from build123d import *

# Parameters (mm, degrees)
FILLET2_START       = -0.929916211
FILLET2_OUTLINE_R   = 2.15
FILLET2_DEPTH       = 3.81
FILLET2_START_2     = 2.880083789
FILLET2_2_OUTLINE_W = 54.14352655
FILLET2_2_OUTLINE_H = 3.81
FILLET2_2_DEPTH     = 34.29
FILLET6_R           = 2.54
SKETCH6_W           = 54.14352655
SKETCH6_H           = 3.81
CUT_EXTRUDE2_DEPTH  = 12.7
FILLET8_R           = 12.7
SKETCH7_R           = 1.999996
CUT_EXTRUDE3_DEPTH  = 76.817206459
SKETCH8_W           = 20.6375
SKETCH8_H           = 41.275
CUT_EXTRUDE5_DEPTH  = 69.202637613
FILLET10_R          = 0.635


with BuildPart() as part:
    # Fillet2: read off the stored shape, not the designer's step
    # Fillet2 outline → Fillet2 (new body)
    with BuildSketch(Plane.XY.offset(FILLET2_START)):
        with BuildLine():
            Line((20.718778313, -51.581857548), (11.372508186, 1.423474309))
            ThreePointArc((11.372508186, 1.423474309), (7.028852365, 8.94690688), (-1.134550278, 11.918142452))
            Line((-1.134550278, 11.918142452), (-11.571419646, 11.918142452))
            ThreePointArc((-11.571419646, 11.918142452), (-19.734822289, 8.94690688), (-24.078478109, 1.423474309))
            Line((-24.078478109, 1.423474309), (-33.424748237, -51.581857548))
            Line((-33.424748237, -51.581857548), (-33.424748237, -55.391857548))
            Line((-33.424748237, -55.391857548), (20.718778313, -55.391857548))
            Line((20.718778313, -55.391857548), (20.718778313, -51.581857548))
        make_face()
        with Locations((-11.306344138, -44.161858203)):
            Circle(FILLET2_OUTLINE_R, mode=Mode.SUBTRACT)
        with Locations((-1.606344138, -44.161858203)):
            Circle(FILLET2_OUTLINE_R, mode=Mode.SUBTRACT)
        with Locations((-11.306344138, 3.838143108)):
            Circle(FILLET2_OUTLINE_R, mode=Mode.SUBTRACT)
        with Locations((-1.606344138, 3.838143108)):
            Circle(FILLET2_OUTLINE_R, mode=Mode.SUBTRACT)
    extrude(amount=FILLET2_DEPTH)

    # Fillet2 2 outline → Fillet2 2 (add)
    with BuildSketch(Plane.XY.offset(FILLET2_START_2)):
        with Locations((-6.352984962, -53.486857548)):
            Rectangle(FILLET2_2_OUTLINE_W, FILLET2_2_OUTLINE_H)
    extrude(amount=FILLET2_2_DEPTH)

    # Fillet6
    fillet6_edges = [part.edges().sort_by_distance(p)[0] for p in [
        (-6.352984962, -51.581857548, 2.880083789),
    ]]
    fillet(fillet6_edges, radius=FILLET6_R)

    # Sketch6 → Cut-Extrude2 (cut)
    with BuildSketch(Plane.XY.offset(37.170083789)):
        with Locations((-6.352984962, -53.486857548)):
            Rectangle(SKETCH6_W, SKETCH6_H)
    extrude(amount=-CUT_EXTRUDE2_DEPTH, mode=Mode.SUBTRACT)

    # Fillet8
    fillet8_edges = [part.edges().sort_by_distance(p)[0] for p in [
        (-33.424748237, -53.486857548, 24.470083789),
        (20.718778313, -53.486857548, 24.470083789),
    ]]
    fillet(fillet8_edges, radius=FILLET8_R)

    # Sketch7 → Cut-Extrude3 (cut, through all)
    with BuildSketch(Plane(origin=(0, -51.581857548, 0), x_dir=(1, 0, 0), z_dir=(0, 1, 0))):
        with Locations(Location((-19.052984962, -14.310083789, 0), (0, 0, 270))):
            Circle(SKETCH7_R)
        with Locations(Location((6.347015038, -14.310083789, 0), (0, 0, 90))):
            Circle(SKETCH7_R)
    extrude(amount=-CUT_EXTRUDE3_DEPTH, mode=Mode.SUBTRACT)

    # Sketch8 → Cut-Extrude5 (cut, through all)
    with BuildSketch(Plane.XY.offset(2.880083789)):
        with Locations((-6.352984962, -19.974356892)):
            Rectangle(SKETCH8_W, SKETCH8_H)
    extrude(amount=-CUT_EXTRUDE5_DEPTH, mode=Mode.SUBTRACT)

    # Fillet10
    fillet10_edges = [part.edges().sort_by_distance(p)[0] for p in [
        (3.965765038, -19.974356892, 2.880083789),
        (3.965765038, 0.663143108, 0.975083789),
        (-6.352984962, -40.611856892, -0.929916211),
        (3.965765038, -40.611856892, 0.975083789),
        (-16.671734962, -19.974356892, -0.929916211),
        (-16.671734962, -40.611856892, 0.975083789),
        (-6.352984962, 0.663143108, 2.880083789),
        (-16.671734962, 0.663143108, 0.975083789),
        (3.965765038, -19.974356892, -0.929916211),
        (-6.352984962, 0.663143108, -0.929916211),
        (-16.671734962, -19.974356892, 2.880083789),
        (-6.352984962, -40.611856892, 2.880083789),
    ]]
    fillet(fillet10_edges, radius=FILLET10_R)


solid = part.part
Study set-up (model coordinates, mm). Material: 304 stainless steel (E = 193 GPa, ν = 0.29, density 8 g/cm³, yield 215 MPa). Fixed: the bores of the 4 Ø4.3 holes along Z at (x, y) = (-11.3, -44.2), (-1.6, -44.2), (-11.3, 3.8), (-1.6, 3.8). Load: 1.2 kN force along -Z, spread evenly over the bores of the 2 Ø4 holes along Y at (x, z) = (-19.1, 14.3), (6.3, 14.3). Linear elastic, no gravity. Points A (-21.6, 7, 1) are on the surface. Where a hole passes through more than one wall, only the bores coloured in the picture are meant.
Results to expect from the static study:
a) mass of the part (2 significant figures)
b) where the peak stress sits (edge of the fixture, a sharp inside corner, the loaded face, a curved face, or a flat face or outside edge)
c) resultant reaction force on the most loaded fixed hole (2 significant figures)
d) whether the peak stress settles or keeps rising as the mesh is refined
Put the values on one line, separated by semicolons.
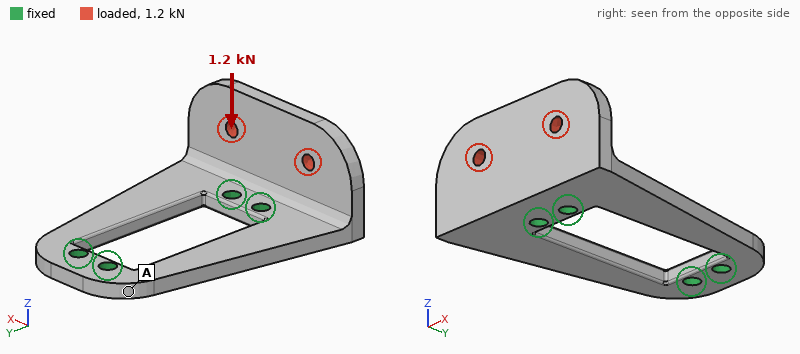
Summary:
93 g; edge of the fixture; 620 N; keeps rising
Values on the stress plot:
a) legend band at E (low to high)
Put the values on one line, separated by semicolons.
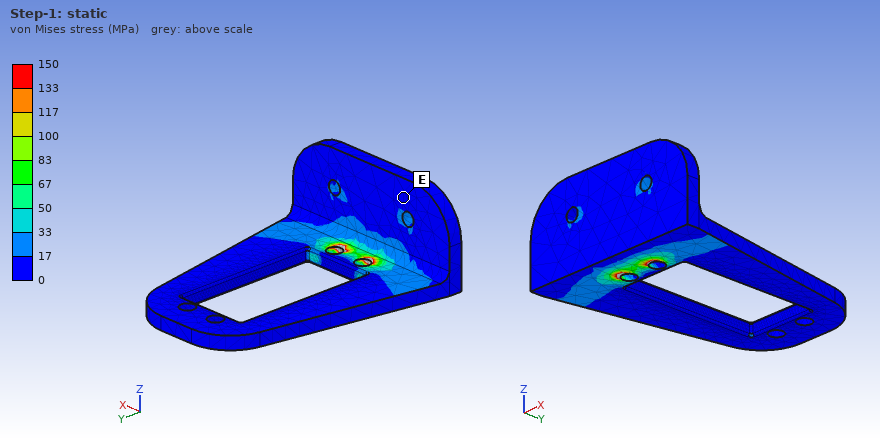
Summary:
0 to 17 MPa
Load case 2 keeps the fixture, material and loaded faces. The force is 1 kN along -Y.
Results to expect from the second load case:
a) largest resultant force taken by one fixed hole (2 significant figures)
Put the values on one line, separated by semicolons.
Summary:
440 N
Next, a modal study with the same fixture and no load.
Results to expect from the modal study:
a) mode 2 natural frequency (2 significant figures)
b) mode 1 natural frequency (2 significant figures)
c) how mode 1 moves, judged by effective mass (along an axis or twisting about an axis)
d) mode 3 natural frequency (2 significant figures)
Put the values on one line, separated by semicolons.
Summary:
4300 Hz; 3600 Hz; along Y; 5400 Hz
